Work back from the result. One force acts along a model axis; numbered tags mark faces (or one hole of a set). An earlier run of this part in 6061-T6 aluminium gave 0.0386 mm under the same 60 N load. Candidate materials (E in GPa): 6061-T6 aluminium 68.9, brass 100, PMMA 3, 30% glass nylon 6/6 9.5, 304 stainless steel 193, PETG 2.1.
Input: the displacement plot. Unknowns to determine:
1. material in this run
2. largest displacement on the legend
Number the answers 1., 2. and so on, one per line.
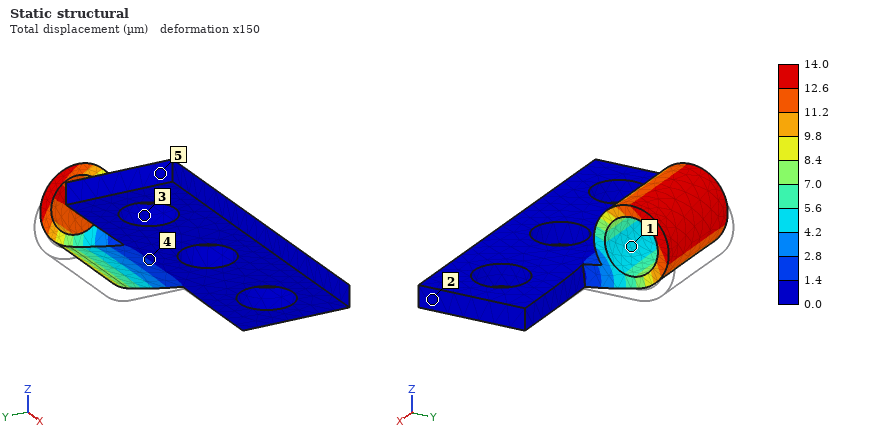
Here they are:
1. 304 stainless steel
2. 14.0 µm
